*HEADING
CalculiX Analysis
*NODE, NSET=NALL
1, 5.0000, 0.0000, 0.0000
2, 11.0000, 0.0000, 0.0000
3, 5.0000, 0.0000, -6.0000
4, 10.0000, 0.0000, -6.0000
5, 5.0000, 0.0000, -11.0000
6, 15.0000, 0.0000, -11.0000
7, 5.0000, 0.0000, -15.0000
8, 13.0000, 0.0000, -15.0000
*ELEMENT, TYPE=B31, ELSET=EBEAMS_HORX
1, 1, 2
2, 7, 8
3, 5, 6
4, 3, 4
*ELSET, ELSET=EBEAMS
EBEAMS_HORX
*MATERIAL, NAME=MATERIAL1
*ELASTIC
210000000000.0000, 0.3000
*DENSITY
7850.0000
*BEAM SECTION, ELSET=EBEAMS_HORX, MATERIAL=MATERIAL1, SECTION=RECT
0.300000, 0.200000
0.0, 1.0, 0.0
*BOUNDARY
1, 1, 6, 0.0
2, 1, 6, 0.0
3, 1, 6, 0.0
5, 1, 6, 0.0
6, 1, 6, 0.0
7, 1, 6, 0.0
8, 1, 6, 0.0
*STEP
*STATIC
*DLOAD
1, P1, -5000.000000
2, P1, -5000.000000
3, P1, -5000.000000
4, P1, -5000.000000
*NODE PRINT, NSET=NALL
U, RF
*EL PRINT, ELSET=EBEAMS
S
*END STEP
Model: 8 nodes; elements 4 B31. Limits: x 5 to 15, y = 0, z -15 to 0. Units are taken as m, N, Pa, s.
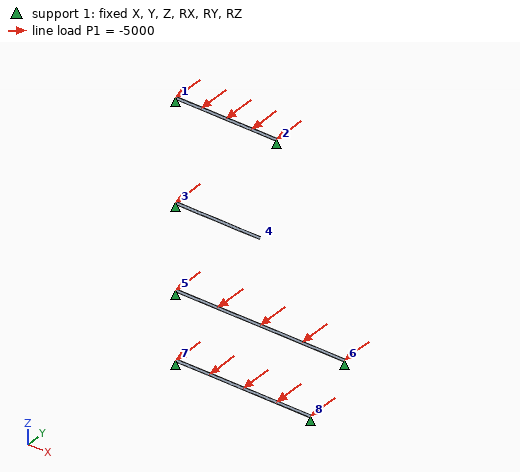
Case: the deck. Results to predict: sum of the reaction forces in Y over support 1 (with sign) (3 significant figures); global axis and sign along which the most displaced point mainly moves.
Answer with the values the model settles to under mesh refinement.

1.45e+05 N
-Y
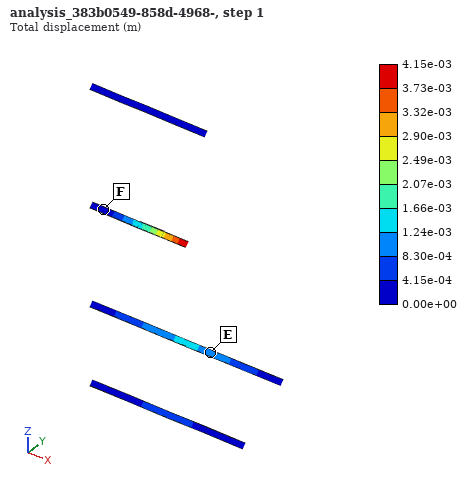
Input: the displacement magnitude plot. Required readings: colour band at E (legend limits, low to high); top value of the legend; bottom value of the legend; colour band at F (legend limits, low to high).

8.30e-04 to 1.24e-03 m
4.15e-03 m
0.00e+00 m
0.00e+00 to 4.15e-04 m
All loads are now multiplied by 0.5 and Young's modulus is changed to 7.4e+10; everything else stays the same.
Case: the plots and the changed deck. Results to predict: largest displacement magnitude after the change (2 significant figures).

0.0059 m
